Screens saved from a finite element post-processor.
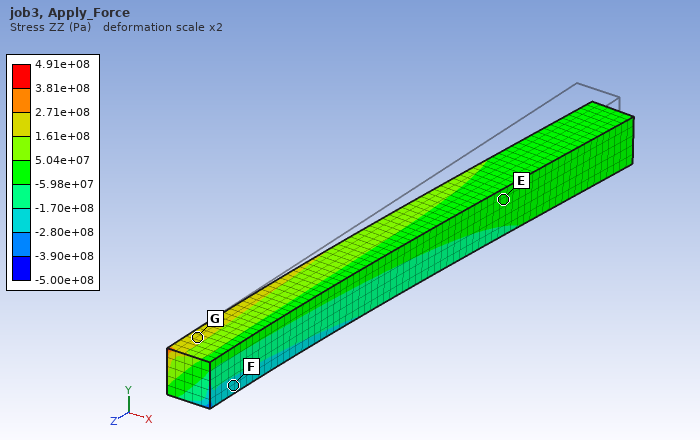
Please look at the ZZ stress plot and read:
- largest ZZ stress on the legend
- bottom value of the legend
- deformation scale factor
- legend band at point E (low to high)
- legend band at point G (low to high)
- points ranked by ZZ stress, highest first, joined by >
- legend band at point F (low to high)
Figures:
4.91e+08 Pa
-5.00e+08 Pa
2
-5.98e+07 to 5.04e+07 Pa
1.61e+08 to 2.71e+08 Pa
G > E > F
-2.80e+08 to -1.70e+08 Pa
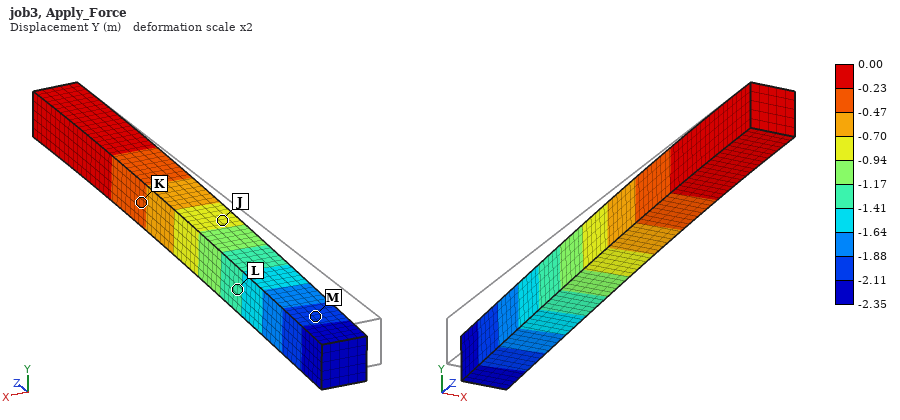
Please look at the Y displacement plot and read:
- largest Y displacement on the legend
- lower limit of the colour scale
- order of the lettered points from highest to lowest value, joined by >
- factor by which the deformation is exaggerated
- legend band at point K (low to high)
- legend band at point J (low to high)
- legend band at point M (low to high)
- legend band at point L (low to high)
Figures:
0.00 m
-2.35 m
K > J > L > M
2
-0.47 to -0.23 m
-0.94 to -0.70 m
-2.11 to -1.88 m
-1.41 to -1.17 m
